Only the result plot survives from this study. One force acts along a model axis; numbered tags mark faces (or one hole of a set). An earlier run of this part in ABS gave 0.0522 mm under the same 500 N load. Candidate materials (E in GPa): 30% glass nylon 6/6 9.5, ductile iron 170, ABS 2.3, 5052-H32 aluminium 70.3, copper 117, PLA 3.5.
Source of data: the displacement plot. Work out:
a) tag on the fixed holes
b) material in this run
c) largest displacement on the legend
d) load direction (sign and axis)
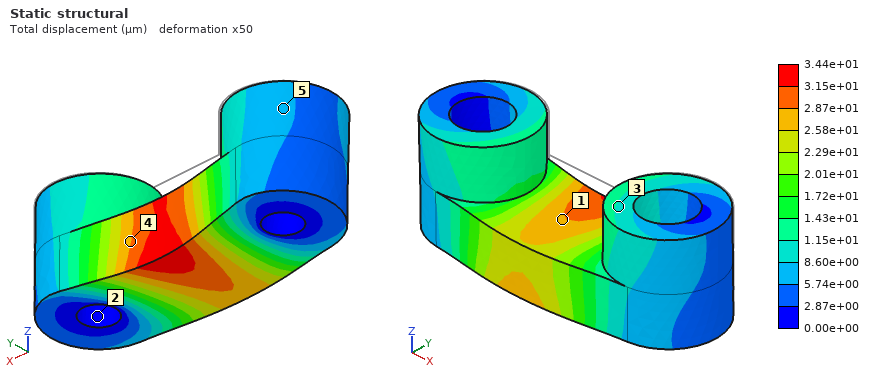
2
PLA
3.44e+01 µm
-Y
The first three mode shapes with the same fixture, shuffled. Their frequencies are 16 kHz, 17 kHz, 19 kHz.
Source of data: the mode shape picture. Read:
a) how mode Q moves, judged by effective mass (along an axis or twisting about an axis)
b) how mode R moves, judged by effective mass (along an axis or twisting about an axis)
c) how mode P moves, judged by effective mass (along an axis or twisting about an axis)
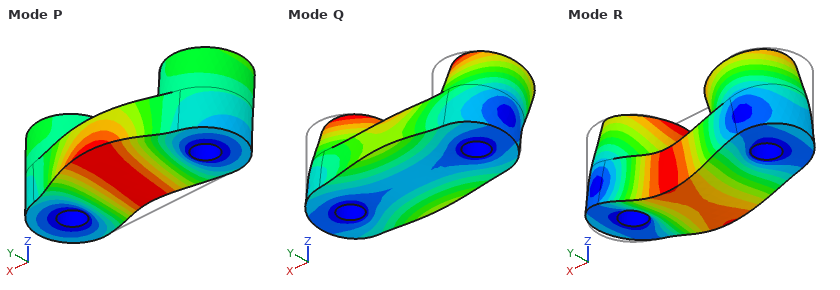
along Y
along Z
along Y
